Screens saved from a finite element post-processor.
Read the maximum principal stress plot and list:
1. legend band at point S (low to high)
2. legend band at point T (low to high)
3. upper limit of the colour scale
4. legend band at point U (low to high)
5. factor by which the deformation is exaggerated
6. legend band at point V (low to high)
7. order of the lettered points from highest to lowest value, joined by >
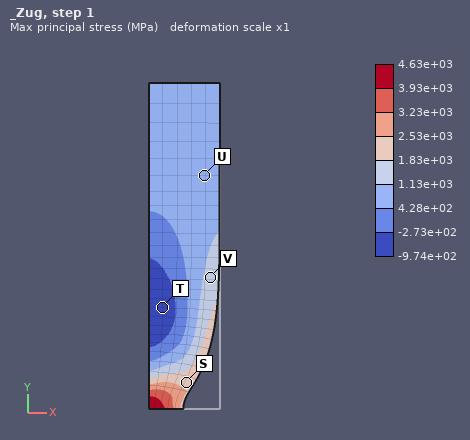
1.83e+03 to 2.53e+03 MPa
-9.74e+02 to -2.73e+02 MPa
4.63e+03 MPa
4.28e+02 to 1.13e+03 MPa
1
1.13e+03 to 1.83e+03 MPa
S > V > U > T
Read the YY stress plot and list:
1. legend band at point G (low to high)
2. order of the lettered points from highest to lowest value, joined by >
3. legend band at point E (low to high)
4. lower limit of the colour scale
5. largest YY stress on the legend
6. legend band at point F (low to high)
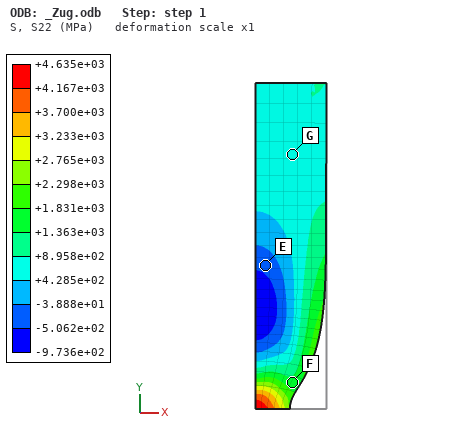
+4.285e+02 to +8.958e+02 MPa
F > G > E
-5.062e+02 to -3.888e+01 MPa
-9.736e+02 MPa
+4.635e+03 MPa
+1.363e+03 to +1.831e+03 MPa
